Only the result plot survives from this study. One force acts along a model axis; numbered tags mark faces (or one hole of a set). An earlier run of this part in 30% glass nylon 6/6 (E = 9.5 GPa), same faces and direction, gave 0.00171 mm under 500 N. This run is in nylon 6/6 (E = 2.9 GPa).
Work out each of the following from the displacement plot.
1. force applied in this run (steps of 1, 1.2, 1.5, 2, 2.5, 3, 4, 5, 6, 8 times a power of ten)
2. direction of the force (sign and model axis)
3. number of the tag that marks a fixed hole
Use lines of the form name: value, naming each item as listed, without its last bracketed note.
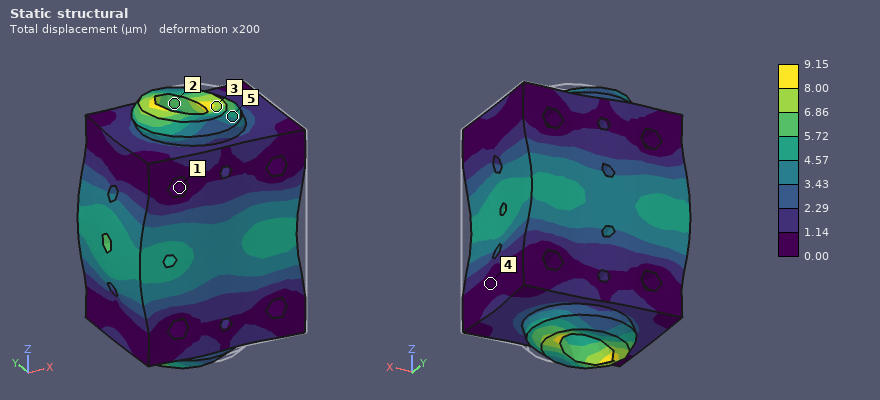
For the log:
force applied in this run: 800 N
direction of the force: -X
number of the tag that marks a fixed hole: 1
